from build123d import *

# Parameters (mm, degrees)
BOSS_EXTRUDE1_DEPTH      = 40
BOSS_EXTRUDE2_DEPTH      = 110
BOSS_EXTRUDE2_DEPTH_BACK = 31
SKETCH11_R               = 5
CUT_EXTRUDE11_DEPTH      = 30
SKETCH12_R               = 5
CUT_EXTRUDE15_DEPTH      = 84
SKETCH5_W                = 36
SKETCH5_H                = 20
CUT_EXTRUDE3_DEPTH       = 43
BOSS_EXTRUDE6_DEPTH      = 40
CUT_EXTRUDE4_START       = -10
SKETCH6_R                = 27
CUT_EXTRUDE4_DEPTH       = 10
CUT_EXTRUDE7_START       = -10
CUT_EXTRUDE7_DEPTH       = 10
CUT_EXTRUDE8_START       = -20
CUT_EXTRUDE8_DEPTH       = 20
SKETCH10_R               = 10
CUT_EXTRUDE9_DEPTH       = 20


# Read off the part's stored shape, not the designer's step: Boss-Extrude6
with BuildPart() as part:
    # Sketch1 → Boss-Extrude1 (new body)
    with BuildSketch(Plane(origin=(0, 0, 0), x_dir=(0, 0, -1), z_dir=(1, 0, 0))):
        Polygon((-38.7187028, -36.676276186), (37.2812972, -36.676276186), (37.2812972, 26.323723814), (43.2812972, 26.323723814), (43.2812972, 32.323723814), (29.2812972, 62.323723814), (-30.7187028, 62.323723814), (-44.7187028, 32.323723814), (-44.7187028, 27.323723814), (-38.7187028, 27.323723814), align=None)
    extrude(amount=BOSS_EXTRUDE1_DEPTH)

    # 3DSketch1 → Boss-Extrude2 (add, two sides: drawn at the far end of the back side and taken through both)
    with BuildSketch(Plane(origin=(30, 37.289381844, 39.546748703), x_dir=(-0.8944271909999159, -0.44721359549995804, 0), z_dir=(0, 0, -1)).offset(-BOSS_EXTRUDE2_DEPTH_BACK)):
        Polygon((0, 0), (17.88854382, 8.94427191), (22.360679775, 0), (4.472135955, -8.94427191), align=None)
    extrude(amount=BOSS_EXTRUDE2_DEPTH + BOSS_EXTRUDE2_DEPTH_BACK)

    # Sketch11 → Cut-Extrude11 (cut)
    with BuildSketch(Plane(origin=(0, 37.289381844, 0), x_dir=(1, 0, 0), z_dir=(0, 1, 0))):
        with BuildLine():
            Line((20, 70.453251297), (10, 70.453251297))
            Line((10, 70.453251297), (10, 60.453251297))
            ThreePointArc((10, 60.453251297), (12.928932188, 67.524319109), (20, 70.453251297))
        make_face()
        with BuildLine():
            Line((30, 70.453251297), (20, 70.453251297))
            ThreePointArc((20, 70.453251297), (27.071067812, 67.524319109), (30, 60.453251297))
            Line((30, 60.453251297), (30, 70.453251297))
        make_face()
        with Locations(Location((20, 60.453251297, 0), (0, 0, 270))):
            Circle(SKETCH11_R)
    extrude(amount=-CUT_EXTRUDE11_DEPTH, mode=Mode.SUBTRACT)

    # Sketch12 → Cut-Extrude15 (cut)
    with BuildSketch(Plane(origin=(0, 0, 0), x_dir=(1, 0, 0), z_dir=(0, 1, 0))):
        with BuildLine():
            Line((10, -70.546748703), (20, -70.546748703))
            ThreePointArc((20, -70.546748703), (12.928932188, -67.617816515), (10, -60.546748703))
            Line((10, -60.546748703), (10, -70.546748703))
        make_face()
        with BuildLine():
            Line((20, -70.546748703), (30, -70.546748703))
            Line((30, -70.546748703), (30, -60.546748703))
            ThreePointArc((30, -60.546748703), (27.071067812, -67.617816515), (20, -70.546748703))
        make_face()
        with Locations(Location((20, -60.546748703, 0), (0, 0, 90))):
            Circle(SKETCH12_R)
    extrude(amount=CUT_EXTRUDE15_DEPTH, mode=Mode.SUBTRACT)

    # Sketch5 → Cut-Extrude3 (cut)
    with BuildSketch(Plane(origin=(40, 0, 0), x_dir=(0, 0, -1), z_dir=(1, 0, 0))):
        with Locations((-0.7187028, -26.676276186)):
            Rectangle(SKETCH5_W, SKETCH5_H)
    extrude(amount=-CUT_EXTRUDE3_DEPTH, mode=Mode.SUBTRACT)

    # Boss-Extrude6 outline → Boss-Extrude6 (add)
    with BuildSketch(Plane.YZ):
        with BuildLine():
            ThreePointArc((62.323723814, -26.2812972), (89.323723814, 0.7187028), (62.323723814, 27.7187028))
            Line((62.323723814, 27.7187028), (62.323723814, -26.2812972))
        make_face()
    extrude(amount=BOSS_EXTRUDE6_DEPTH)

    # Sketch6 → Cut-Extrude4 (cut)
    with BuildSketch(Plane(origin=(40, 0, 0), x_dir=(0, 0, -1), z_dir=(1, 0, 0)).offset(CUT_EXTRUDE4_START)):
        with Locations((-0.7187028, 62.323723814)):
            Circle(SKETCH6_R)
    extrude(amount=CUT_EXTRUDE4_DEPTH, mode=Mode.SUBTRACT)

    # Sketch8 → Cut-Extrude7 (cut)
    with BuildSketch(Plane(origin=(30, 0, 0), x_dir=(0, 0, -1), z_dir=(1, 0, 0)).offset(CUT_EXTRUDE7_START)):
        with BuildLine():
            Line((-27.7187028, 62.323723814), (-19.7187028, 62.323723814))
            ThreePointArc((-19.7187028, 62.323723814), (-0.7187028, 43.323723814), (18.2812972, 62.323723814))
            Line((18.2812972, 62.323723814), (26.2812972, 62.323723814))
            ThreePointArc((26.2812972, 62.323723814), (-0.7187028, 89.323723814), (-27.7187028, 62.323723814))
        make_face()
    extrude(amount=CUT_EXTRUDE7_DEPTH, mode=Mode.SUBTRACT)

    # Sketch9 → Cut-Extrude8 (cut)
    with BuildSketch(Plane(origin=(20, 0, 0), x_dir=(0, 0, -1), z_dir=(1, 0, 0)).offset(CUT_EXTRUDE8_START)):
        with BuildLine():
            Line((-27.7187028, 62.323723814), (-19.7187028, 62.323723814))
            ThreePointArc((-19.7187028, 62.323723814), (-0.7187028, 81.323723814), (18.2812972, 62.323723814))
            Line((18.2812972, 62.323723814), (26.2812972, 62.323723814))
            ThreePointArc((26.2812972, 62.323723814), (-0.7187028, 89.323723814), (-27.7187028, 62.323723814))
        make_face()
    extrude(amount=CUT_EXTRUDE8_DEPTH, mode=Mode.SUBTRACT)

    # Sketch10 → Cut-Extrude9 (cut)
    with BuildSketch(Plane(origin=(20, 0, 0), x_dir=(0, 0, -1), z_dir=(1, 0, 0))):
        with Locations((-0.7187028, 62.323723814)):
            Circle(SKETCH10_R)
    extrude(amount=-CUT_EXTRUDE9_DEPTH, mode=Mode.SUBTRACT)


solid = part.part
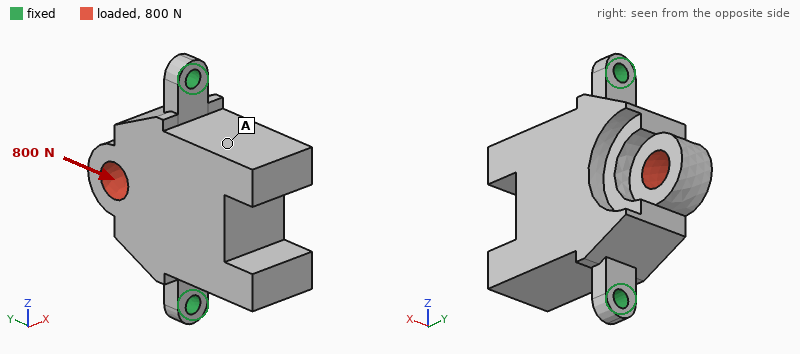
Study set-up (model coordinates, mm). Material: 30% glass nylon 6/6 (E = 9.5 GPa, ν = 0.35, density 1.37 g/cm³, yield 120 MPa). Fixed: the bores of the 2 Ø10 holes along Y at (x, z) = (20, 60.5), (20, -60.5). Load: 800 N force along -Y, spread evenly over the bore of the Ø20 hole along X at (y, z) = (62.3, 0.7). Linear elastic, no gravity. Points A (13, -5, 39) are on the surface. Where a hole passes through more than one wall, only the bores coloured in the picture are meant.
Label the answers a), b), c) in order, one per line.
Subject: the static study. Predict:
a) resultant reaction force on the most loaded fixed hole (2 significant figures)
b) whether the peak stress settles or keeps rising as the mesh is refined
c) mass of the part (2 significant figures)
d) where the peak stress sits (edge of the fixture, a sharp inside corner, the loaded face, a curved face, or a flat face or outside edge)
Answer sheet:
a) 410 N
b) keeps rising
c) 370 g
d) edge of the fixture
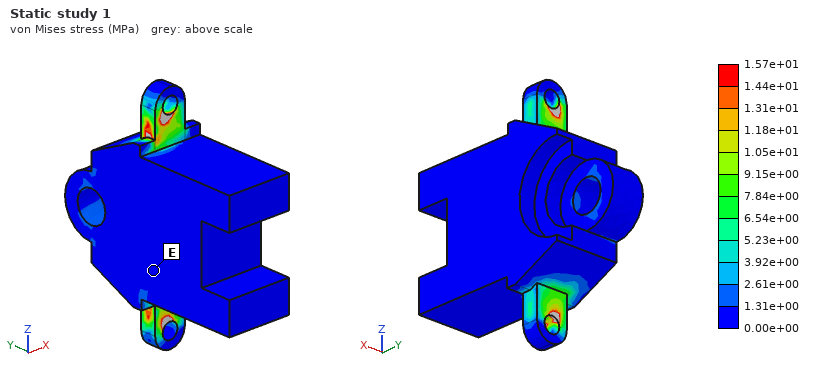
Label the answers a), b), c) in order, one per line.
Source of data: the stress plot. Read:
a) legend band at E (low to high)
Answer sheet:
a) 0.00e+00 to 1.31e+00 MPa
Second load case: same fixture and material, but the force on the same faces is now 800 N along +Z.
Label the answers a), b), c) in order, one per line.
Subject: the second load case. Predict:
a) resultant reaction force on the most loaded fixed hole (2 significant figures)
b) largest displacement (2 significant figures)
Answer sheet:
a) 490 N
b) 30 µm
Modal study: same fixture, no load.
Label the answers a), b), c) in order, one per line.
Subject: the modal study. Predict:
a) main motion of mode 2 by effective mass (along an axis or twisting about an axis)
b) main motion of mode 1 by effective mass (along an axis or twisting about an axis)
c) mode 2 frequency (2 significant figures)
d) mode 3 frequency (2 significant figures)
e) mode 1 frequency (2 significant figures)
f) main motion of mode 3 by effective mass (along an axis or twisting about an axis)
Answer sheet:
a) along Y
b) along X
c) 1400 Hz
d) 1700 Hz
e) 370 Hz
f) along Z
